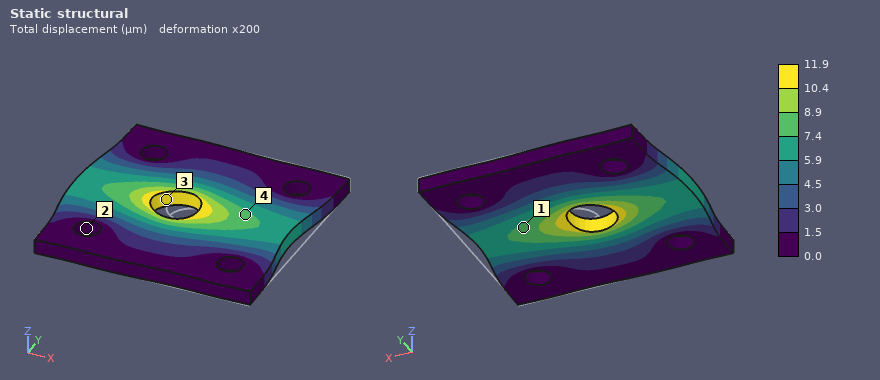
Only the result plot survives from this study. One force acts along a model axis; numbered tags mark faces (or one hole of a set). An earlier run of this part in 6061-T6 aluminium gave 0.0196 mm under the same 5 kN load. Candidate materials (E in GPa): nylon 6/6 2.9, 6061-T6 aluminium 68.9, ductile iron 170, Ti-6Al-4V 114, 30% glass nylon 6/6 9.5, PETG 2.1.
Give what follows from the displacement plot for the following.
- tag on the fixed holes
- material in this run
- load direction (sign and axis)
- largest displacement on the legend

2
Ti-6Al-4V
-X
11.9 µm
